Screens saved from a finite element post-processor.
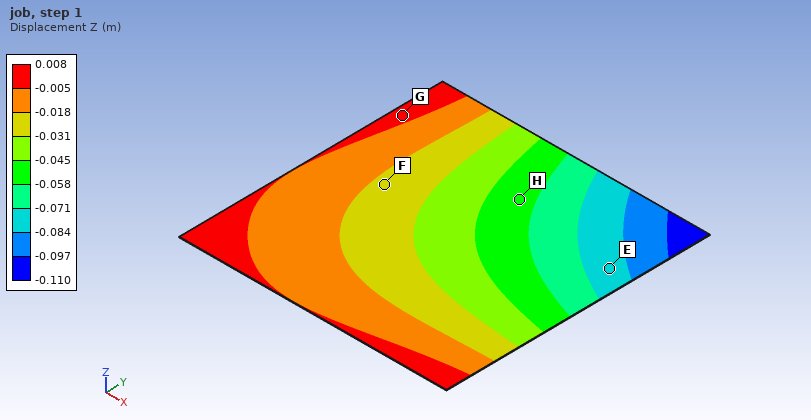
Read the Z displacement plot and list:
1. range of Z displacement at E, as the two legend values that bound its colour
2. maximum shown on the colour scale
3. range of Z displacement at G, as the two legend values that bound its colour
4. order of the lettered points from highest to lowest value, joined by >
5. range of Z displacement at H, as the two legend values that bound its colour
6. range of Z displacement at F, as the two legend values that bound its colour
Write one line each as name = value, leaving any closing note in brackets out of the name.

range of Z displacement at E, as the two legend values that bound its colour = -0.084 to -0.071 m
maximum shown on the colour scale = 0.008 m
range of Z displacement at G, as the two legend values that bound its colour = -0.005 to 0.008 m
order of the lettered points from highest to lowest value, joined by > = G > F > H > E
range of Z displacement at H, as the two legend values that bound its colour = -0.058 to -0.045 m
range of Z displacement at F, as the two legend values that bound its colour = -0.031 to -0.018 m
